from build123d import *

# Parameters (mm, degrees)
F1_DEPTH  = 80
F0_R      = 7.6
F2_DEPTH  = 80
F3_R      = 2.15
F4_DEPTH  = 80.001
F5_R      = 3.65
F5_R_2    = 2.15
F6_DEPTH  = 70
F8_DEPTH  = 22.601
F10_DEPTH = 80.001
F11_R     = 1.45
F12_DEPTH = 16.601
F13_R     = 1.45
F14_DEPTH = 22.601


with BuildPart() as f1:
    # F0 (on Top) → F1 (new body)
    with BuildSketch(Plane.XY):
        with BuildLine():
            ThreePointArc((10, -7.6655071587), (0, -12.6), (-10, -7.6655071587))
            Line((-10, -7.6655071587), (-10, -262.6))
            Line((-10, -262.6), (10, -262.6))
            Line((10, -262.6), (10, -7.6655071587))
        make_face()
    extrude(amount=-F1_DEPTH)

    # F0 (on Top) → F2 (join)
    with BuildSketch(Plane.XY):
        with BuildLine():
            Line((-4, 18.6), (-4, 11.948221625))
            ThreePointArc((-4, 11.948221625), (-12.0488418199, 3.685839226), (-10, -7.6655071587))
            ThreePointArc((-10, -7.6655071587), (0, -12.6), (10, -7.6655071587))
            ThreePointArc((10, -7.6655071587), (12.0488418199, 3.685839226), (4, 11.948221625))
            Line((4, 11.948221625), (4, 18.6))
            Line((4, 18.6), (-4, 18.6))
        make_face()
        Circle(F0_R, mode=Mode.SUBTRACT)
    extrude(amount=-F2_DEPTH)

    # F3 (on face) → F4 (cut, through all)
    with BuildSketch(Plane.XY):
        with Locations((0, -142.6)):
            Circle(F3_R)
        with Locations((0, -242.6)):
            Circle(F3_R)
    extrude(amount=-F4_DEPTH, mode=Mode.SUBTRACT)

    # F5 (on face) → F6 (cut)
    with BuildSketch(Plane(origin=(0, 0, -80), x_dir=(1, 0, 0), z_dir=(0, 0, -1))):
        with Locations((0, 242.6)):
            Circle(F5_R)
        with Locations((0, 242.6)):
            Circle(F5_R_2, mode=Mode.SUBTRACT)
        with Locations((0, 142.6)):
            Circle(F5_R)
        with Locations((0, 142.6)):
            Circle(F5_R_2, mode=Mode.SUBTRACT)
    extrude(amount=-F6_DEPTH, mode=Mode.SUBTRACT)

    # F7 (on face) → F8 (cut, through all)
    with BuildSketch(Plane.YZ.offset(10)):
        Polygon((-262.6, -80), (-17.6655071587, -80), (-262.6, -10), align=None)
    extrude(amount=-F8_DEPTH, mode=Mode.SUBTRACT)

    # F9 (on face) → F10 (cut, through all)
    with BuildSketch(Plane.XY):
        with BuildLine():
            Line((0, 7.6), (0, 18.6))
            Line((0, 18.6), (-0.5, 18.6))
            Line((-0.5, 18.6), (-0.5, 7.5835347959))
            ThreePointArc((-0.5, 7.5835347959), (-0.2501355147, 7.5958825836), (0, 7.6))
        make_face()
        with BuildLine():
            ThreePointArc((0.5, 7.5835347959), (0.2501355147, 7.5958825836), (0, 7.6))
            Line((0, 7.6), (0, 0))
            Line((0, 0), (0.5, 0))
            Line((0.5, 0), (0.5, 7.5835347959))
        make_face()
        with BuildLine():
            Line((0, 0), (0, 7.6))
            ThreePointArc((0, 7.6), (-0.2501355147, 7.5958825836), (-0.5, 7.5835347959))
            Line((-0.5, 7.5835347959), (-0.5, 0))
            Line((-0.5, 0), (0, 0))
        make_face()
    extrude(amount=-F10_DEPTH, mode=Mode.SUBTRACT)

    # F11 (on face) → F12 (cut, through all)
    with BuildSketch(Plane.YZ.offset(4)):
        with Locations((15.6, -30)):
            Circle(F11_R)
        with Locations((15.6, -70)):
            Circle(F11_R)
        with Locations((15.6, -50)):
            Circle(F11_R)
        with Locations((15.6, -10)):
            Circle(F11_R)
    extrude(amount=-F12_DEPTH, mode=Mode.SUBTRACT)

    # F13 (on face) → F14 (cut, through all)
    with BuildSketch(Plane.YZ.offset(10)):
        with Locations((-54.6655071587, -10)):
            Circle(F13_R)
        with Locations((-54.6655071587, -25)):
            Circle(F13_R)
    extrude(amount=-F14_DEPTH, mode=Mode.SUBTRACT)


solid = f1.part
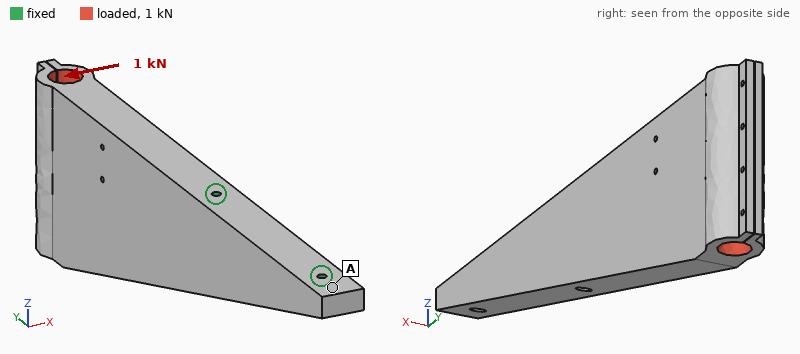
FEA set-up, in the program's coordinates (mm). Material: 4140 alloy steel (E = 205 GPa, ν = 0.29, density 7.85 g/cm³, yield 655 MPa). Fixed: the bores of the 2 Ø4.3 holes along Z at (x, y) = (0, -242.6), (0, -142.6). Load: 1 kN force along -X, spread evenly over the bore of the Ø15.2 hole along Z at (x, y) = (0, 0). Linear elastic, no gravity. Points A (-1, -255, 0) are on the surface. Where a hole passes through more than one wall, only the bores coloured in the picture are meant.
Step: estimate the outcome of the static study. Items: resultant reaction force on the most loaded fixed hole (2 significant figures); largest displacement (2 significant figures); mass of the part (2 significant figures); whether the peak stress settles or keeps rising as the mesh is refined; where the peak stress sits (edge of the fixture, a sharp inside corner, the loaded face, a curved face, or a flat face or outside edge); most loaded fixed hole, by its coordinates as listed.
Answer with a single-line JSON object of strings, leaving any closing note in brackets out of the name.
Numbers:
{"resultant reaction force on the most loaded fixed hole": "2.2 kN", "largest displacement": "0.33 mm", "mass of the part": "2.0 kg", "whether the peak stress settles or keeps rising as the mesh is refined": "keeps rising", "where the peak stress sits": "edge of the fixture", "most loaded fixed hole, by its coordinates as listed": "(0, -142.6)"}
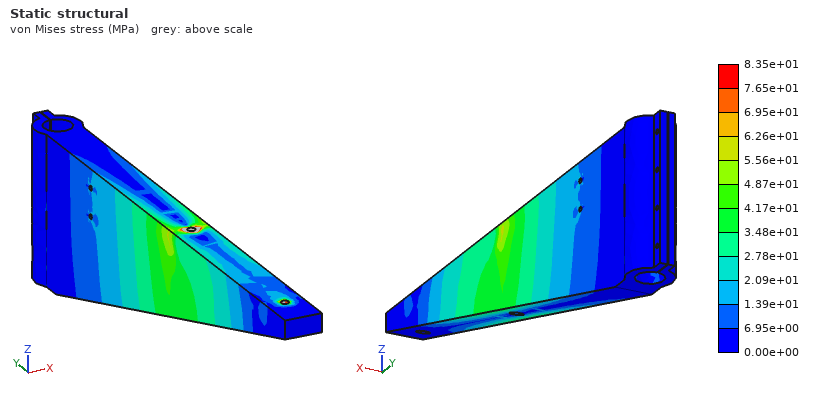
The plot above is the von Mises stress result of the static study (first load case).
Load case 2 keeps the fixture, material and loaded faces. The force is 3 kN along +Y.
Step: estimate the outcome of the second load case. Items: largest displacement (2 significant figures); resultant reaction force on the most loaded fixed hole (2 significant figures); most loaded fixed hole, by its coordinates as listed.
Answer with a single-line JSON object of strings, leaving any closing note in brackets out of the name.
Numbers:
{"largest displacement": "39 µm", "resultant reaction force on the most loaded fixed hole": "2.4 kN", "most loaded fixed hole, by its coordinates as listed": "(0, -242.6)"}
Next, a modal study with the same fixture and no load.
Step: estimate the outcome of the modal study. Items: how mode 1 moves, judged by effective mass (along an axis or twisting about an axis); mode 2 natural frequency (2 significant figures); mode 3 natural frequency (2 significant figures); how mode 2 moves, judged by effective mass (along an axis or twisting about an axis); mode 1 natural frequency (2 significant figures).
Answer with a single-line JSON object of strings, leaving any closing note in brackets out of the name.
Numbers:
{"how mode 1 moves, judged by effective mass": "along X", "mode 2 natural frequency": "820 Hz", "mode 3 natural frequency": "1400 Hz", "how mode 2 moves, judged by effective mass": "along Z", "mode 1 natural frequency": "400 Hz"}
